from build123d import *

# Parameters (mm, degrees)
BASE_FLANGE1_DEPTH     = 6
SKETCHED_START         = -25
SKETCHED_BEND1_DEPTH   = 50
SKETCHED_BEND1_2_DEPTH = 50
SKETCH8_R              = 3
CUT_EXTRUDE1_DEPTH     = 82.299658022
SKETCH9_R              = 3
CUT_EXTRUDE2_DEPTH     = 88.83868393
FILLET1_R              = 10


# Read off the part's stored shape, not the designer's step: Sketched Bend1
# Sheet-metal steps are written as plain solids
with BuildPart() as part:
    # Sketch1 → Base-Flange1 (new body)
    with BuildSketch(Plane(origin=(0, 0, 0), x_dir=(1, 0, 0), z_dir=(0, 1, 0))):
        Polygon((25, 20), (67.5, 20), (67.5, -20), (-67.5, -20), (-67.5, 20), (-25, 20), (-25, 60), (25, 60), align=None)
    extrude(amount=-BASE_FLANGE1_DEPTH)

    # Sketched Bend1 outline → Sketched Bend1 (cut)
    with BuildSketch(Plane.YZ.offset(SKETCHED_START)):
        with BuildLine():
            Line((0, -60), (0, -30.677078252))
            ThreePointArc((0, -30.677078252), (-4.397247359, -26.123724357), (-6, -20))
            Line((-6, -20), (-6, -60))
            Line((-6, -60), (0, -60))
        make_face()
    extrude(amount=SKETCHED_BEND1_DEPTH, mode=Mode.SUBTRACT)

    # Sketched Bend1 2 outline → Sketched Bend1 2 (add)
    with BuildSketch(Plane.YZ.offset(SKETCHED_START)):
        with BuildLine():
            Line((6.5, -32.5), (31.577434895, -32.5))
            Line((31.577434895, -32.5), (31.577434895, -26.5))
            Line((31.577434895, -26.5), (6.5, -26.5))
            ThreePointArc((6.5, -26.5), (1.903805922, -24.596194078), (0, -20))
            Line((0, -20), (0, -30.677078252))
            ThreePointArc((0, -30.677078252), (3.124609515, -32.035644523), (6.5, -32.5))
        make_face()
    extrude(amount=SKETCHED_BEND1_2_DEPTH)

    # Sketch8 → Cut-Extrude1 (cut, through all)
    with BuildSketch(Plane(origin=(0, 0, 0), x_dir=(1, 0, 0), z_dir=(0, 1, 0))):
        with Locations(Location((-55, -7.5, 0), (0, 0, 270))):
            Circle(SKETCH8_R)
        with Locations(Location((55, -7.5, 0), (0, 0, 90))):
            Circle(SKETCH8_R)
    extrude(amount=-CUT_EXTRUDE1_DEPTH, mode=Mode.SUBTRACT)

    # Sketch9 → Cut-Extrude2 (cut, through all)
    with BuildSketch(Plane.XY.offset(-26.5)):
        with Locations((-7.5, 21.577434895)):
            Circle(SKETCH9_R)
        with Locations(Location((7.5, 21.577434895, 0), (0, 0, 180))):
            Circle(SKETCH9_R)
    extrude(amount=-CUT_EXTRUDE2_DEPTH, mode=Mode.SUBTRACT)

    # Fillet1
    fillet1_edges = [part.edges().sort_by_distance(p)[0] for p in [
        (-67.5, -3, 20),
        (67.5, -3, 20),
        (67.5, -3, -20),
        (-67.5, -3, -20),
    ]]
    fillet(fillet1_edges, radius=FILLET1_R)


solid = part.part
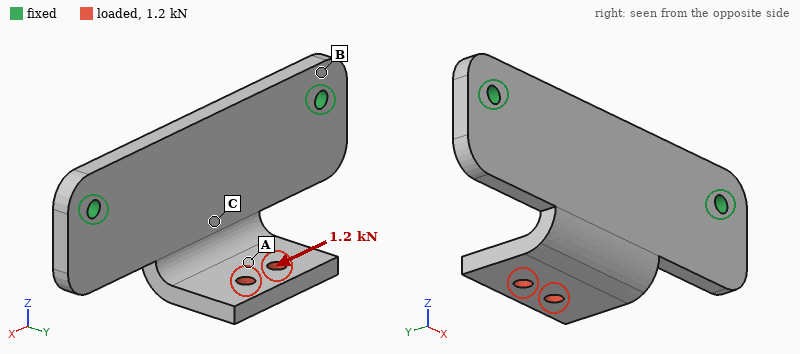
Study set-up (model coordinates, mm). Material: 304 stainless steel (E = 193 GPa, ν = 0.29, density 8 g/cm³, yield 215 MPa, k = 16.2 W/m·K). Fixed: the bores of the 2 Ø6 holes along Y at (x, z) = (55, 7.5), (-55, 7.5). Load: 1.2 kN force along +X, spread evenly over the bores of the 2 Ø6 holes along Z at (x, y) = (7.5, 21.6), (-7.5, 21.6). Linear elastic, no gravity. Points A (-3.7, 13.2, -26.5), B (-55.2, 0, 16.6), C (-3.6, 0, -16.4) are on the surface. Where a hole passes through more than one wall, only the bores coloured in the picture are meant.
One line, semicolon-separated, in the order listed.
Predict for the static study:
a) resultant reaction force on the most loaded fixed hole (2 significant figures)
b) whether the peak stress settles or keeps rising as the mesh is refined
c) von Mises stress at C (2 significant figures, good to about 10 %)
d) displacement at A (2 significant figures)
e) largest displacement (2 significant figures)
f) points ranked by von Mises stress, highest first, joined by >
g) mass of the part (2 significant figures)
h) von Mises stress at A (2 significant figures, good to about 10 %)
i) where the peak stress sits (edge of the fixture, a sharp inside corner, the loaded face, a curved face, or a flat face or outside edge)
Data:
800 N; keeps rising; 39 MPa; 31 µm; 77 µm; C > A > B; 350 g; 22 MPa; a sharp inside corner
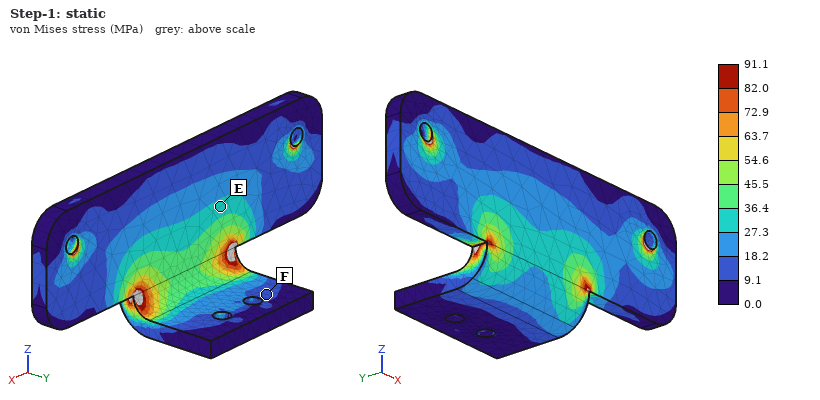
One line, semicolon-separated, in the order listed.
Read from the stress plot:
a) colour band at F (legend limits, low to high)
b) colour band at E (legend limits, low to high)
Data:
9.1 to 18.2 MPa; 27.3 to 36.4 MPa
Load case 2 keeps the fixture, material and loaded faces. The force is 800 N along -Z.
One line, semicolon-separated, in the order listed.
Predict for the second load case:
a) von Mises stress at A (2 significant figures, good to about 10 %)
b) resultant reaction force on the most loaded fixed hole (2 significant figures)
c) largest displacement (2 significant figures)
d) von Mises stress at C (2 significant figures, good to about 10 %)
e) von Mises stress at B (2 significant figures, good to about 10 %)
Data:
25 MPa; 510 N; 0.19 mm; 49 MPa; 22 MPa
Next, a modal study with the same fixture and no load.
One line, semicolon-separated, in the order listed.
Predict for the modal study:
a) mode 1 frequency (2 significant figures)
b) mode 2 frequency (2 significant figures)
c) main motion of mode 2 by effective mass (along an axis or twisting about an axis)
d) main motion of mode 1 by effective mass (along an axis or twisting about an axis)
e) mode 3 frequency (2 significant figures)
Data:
1100 Hz; 2300 Hz; along Y; along Y; 2700 Hz
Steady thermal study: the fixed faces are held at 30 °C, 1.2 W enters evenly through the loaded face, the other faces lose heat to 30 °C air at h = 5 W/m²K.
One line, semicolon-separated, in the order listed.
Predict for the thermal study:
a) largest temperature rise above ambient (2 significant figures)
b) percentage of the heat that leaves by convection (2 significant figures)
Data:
14 K; 35 %
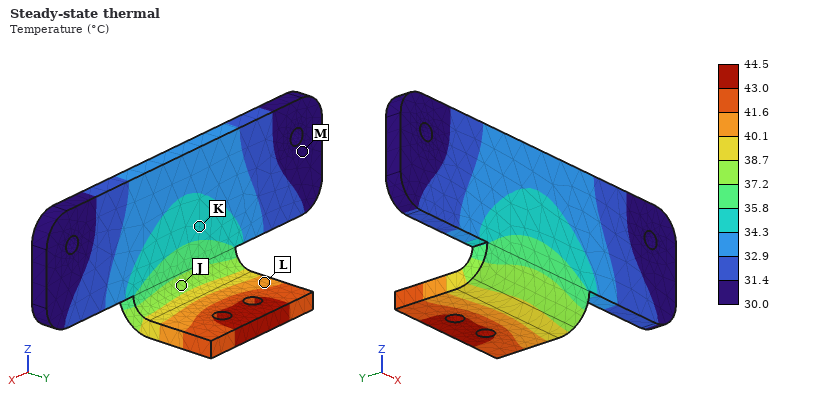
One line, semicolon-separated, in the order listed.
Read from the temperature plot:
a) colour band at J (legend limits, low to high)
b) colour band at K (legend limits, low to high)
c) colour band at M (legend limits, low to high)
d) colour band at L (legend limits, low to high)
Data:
37.2 to 38.7 °C; 34.3 to 35.8 °C; 30.0 to 31.4 °C; 40.1 to 41.6 °C
